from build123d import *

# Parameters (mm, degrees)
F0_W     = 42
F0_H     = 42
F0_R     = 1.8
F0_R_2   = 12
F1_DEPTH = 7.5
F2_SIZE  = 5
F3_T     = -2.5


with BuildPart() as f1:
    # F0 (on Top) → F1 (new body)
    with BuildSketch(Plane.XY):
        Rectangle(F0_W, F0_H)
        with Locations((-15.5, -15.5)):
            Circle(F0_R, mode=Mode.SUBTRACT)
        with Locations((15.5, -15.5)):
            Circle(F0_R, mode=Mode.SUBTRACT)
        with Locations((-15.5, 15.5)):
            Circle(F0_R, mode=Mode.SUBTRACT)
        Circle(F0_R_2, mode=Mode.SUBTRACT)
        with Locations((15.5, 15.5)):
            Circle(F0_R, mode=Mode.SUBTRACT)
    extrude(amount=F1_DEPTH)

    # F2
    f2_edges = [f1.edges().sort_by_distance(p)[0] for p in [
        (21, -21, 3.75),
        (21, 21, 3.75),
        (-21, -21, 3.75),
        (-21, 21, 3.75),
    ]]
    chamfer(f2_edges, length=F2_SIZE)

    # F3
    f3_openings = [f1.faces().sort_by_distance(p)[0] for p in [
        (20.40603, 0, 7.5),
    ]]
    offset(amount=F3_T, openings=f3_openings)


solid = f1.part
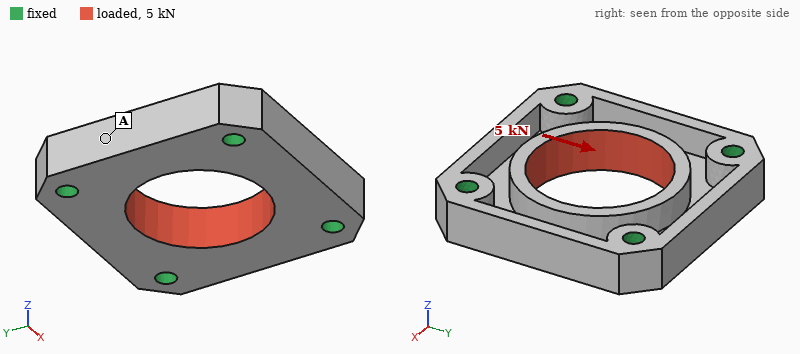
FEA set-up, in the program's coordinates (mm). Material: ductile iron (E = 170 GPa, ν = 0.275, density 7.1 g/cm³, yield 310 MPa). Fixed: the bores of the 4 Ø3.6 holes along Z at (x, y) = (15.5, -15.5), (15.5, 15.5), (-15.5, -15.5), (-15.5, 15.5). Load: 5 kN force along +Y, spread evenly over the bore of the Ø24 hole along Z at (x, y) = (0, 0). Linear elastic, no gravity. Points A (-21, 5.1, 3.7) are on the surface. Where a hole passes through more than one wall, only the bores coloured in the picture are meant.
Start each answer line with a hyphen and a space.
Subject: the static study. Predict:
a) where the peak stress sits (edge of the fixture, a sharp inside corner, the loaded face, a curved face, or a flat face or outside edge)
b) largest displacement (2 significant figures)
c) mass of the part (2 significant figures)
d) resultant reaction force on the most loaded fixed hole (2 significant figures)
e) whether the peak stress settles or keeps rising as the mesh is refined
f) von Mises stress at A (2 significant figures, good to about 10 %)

- edge of the fixture
- 10 µm
- 47 g
- 1.3 kN
- keeps rising
- 14 MPa
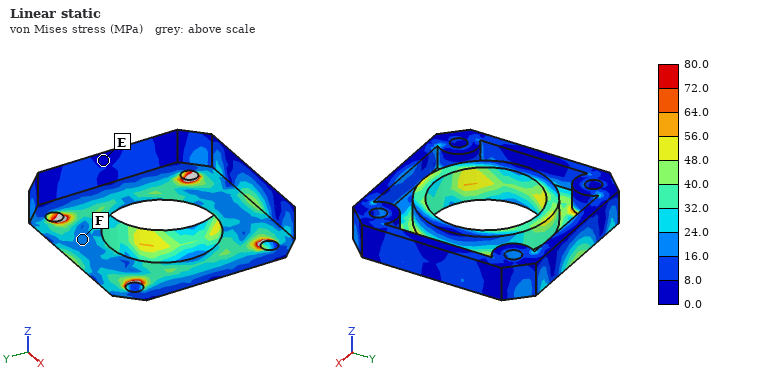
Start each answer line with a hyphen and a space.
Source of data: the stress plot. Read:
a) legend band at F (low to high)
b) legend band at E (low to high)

- 16.0 to 24.0 MPa
- 0.0 to 8.0 MPa
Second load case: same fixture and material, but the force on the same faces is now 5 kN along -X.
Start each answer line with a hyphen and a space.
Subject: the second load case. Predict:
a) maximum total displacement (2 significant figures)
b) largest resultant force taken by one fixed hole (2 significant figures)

- 10 µm
- 1.3 kN
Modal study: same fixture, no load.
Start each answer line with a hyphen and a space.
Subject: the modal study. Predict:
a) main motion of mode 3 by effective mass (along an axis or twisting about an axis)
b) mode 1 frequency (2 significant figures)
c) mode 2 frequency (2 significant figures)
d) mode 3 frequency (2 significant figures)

- twisting about X
- 22 kHz
- 23 kHz
- 25 kHz
